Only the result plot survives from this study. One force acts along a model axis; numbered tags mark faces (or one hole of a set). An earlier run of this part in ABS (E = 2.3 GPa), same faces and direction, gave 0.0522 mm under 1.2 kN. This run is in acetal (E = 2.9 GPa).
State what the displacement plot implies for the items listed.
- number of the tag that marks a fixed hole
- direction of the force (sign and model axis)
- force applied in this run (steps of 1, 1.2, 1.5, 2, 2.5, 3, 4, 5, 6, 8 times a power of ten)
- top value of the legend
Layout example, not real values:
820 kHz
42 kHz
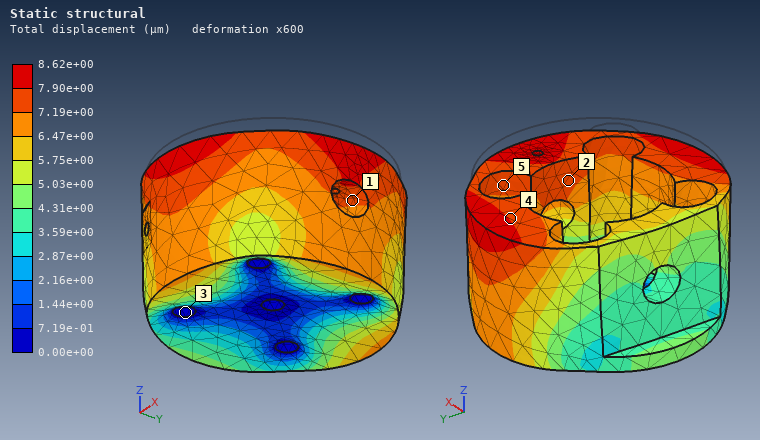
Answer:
3
-Z
250 N
8.62e+00 µm
